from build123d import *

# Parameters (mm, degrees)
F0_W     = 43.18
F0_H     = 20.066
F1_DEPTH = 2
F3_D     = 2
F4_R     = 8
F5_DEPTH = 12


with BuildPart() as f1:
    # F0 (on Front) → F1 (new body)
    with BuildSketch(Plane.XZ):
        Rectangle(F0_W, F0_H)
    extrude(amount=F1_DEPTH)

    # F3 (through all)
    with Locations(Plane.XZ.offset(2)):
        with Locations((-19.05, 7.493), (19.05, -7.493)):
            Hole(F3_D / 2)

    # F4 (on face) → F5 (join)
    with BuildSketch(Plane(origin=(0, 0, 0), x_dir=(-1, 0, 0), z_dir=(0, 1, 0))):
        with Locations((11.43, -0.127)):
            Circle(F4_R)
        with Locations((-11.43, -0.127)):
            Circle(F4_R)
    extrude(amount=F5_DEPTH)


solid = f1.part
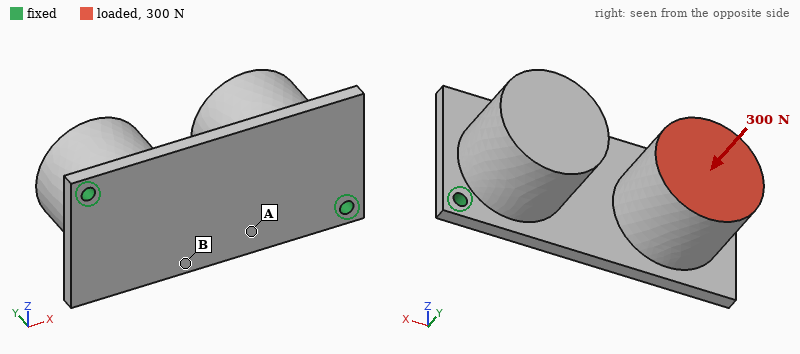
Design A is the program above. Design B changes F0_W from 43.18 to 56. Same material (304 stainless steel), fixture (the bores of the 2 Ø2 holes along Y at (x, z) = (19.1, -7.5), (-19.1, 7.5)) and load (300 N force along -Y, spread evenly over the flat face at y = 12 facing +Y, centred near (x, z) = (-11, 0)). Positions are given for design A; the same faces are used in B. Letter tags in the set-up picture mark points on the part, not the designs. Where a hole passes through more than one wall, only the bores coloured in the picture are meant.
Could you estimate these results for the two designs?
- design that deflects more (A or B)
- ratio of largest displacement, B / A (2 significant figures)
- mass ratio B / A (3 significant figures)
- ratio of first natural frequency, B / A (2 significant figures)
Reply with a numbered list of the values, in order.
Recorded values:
1. A
2. 0.91
3. 1.08
4. 1.0
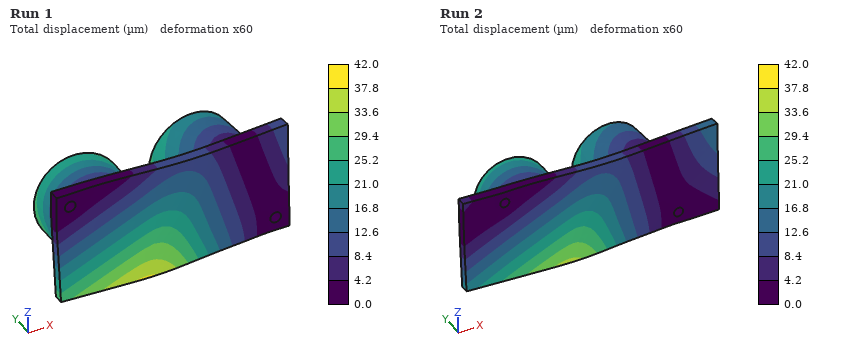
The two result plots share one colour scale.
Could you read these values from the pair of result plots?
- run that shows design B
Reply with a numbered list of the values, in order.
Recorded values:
1. Run 2
